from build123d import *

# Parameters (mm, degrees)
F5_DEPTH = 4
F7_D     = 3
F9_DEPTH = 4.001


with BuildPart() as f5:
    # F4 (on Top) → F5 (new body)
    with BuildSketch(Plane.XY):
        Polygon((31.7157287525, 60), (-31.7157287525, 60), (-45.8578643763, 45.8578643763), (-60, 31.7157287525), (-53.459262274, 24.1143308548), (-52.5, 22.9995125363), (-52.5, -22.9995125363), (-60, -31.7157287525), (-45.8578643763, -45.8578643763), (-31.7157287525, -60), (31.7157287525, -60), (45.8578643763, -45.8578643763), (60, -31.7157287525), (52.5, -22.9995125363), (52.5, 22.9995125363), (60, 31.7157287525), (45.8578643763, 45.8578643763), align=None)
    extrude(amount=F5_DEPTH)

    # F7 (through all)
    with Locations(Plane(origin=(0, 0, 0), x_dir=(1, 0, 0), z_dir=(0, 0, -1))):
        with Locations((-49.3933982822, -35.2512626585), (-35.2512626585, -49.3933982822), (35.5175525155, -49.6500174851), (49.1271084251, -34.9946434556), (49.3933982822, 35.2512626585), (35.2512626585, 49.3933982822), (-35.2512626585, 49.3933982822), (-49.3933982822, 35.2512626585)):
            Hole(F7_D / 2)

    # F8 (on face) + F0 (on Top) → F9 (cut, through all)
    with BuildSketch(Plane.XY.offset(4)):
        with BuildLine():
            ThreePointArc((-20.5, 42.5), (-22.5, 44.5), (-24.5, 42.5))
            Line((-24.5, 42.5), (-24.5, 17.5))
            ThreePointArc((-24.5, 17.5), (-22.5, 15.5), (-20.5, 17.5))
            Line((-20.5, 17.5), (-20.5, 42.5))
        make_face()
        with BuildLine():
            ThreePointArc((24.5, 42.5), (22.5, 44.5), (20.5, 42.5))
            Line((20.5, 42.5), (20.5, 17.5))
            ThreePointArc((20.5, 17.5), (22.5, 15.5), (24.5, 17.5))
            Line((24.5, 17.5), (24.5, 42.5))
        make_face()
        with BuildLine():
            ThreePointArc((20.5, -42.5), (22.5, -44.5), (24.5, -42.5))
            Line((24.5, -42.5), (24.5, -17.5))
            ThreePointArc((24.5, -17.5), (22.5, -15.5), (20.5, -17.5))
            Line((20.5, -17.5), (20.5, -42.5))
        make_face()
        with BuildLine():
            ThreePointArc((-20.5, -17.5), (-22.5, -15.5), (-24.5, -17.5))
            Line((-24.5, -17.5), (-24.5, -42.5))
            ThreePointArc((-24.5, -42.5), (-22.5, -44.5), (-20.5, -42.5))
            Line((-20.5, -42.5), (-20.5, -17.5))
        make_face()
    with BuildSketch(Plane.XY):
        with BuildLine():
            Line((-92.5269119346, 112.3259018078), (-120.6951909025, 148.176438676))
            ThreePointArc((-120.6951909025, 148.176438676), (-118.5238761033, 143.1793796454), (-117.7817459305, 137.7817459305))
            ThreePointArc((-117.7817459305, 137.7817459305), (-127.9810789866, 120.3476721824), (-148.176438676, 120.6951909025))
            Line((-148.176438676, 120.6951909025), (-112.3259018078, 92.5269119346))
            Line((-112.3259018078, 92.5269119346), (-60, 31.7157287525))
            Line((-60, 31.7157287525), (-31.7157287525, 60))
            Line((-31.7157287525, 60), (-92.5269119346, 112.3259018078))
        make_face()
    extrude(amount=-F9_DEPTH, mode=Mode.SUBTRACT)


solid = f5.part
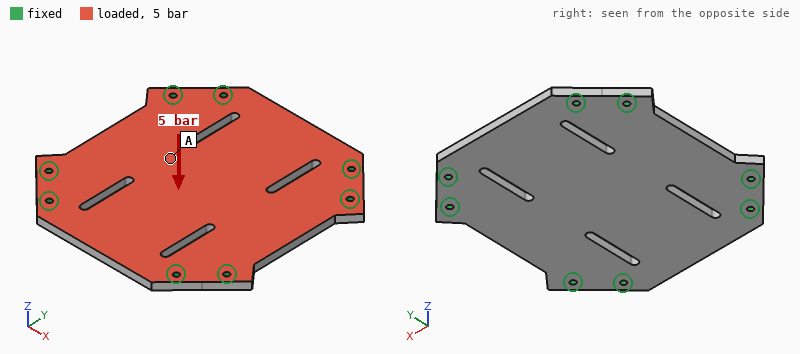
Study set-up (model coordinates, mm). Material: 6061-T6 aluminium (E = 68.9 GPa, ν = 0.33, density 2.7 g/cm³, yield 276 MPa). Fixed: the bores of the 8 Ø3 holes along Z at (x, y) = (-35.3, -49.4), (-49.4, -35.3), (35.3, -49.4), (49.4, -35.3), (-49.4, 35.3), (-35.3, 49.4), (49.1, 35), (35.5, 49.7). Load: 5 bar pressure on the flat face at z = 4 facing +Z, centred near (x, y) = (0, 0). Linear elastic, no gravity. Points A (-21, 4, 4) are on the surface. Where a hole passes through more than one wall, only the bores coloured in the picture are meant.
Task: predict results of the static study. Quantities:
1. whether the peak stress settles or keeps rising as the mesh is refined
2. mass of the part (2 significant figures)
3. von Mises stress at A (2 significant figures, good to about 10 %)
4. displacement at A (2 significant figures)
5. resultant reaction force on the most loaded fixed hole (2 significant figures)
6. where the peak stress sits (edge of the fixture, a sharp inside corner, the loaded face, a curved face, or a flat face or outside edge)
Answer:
keeps rising
120 g
59 MPa
0.37 mm
800 N
edge of the fixture
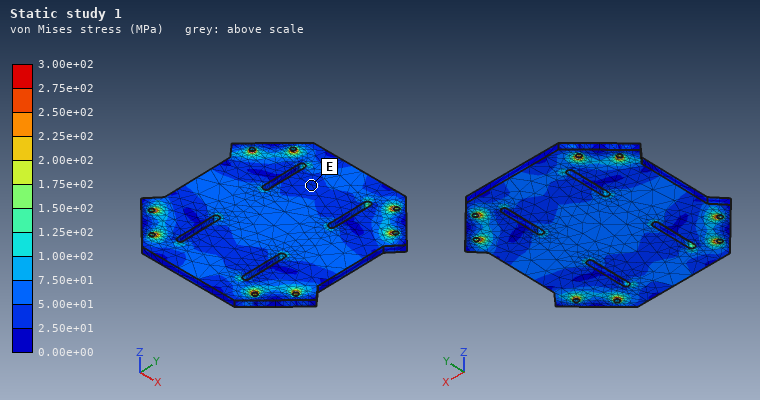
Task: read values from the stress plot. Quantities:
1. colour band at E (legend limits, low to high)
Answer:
2.50e+01 to 5.00e+01 MPa
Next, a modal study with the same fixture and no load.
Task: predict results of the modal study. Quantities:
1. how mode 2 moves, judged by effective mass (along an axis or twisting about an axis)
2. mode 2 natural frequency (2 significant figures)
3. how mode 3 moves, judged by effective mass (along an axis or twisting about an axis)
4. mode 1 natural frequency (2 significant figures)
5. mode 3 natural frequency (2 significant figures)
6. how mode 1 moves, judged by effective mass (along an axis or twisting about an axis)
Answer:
twisting about X
3600 Hz
twisting about Y
2000 Hz
3700 Hz
along Z
